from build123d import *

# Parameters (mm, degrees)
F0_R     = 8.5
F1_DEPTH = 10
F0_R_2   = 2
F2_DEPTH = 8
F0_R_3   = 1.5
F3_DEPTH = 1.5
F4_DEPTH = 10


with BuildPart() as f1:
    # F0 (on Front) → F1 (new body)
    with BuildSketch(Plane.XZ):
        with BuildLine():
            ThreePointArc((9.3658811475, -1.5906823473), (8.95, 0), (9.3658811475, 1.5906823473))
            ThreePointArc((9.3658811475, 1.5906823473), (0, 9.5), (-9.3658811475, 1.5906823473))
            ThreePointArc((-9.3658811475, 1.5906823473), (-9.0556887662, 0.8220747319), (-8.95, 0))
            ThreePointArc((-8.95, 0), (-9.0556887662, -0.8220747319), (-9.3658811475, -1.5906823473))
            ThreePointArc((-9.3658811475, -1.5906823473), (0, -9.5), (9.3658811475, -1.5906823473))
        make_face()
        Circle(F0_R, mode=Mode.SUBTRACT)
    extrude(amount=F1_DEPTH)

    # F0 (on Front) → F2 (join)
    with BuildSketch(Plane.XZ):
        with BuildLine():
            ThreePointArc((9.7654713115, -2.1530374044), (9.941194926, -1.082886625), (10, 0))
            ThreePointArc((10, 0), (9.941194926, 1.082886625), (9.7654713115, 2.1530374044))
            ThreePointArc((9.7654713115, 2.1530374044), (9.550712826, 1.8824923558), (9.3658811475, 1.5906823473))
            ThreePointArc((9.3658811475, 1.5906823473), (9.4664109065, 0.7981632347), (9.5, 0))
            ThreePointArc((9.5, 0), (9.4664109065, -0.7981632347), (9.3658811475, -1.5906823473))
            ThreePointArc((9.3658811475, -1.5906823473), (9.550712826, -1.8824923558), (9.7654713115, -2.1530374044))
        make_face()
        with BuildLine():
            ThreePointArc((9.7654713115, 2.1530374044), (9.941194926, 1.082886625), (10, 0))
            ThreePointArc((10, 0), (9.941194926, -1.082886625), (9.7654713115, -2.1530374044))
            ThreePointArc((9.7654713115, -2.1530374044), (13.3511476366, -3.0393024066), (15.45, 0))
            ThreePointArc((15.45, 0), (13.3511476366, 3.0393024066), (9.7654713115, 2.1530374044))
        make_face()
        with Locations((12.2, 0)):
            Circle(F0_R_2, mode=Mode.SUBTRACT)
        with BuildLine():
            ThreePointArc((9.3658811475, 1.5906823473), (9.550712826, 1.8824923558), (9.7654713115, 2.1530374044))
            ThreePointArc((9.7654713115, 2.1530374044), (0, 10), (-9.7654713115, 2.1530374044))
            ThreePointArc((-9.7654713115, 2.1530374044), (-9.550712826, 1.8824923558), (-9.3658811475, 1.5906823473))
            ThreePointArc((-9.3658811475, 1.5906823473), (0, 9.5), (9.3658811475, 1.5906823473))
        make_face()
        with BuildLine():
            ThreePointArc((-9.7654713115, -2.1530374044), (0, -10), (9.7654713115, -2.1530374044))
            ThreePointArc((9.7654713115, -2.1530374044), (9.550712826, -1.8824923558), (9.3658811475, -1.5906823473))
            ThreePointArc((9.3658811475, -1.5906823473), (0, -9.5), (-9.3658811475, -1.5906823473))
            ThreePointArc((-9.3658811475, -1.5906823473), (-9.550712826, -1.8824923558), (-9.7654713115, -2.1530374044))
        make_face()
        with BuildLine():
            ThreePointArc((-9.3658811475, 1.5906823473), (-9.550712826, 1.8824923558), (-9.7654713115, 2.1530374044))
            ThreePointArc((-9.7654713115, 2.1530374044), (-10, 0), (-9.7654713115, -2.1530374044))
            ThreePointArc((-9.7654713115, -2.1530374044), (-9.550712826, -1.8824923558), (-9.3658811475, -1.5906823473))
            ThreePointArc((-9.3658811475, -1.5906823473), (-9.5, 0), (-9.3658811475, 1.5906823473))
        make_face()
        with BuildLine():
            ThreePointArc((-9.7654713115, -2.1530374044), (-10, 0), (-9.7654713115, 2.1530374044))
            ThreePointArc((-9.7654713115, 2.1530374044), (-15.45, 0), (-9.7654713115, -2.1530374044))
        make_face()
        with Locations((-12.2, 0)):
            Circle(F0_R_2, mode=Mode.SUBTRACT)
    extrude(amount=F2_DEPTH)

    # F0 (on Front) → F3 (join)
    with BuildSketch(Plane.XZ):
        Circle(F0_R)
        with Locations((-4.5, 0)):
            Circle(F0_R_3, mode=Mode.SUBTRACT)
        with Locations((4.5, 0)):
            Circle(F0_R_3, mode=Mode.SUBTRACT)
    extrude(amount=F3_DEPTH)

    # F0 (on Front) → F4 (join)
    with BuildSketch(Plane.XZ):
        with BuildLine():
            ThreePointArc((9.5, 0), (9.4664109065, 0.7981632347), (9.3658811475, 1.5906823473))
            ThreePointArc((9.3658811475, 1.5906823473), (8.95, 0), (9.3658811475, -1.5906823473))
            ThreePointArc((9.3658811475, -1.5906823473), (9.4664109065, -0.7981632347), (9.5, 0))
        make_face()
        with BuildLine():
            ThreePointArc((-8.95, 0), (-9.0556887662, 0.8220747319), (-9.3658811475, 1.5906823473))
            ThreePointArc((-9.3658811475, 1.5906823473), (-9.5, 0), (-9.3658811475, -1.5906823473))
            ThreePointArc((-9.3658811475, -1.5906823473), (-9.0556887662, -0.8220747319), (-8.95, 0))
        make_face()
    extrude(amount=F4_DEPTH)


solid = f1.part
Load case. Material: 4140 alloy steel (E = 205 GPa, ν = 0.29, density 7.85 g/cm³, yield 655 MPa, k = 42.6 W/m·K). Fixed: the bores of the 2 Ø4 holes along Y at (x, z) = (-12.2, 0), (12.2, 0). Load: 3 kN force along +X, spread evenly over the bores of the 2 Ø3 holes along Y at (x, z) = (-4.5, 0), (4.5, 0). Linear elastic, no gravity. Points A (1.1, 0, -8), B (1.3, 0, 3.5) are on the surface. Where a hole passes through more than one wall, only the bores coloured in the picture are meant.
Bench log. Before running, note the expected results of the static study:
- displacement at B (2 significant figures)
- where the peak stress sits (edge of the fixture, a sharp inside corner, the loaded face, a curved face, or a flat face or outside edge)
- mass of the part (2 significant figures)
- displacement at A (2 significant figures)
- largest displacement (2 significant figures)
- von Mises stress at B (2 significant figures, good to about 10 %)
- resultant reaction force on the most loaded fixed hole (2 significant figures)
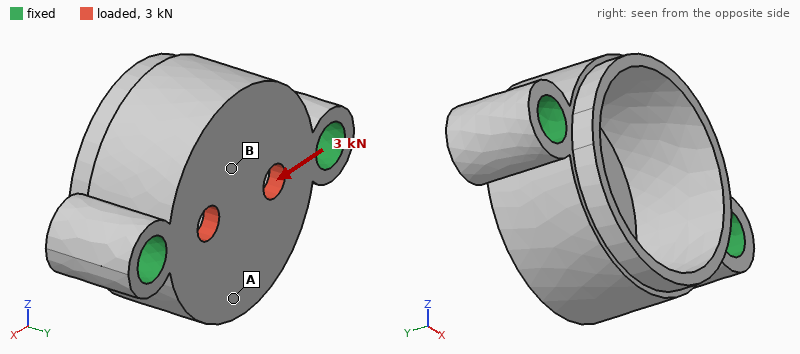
4.2 µm
the loaded face
11 g
2.8 µm
7.0 µm
39 MPa
1.5 kN
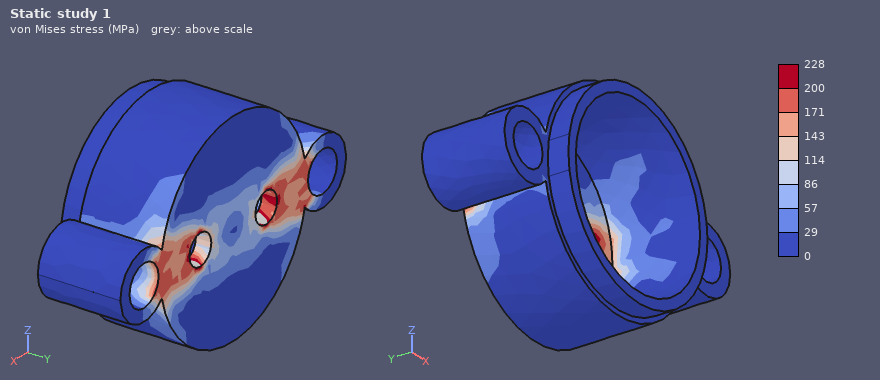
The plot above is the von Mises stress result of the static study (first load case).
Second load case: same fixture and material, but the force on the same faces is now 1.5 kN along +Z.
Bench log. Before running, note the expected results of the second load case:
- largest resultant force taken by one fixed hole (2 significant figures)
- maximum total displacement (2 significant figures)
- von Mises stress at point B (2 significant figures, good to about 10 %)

750 N
5.1 µm
13 MPa
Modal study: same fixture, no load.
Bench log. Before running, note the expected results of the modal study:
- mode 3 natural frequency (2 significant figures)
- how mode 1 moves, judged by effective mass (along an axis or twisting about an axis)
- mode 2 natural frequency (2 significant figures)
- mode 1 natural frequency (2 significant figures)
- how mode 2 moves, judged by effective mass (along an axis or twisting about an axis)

32 kHz
twisting about X
29 kHz
27 kHz
along Y
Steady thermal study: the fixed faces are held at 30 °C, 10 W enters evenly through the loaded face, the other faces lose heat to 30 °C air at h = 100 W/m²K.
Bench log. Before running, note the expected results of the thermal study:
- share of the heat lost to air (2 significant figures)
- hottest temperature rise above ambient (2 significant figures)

21 %
39 K
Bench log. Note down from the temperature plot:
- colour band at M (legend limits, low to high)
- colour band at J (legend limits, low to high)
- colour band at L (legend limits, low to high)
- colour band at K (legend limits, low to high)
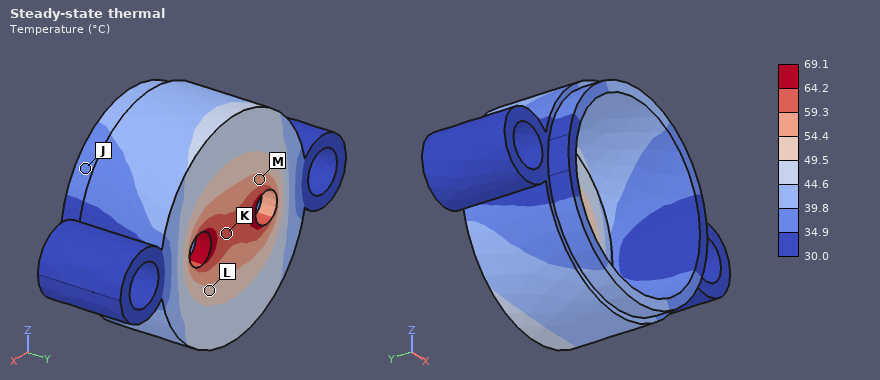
54.4 to 59.3 °C
34.9 to 39.8 °C
49.5 to 54.4 °C
59.3 to 64.2 °C
